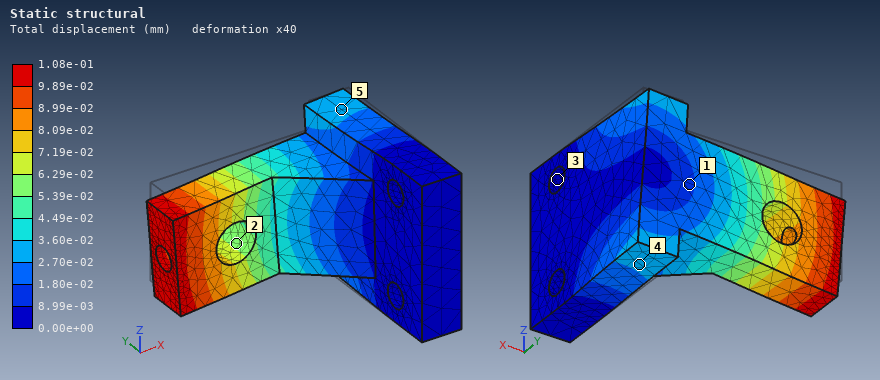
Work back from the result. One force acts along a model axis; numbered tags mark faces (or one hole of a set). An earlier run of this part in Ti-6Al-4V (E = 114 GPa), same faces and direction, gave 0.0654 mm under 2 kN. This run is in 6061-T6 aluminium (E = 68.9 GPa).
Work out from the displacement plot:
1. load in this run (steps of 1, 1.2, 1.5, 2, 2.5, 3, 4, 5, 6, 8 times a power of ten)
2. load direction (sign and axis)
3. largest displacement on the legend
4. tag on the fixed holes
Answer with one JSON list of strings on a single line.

["2 kN", "-Z", "1.08e-01 mm", "3"]
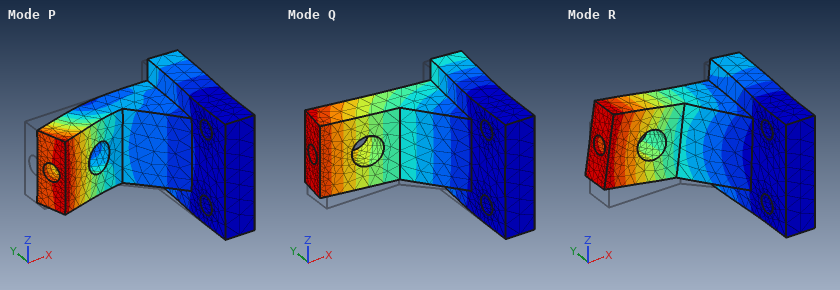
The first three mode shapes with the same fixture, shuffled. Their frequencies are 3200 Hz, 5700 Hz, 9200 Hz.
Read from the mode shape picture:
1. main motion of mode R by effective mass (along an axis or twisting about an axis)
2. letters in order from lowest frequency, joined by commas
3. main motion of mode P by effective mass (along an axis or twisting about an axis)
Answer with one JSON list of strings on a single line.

["along Z", "Q, R, P", "along X"]
